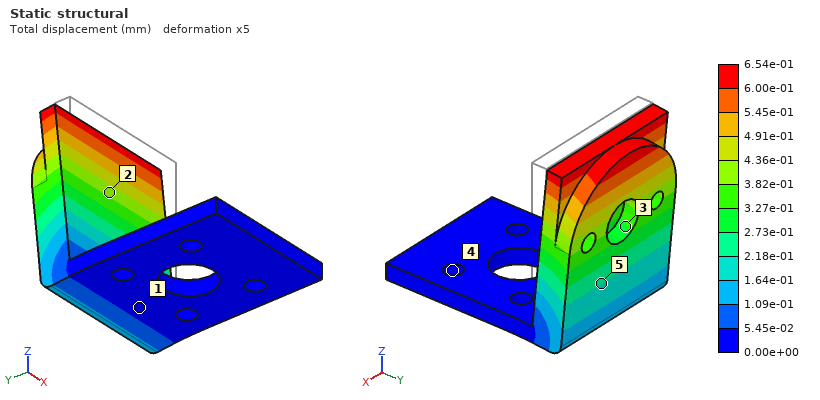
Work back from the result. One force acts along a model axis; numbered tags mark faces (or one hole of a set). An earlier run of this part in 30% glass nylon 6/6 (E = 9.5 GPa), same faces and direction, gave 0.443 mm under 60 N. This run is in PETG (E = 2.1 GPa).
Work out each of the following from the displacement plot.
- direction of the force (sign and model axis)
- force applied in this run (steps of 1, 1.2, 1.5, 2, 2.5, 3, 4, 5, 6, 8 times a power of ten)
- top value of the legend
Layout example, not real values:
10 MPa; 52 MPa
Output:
+Y; 20 N; 6.54e-01 mm
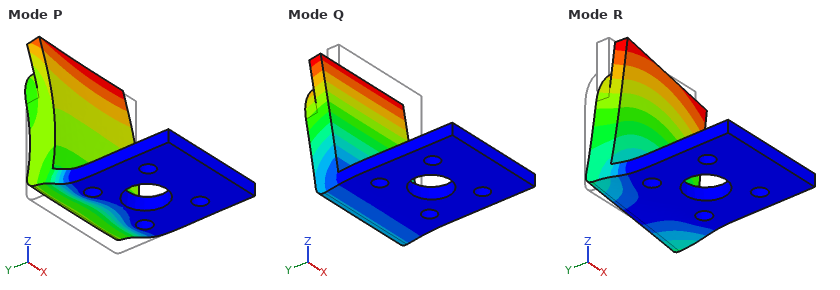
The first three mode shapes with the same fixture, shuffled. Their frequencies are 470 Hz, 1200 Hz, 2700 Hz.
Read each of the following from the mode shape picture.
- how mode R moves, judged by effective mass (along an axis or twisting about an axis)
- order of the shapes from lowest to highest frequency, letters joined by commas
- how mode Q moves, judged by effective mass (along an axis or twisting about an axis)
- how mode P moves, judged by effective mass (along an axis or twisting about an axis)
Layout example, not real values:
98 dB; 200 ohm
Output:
along X; Q, R, P; along Y; along Z
